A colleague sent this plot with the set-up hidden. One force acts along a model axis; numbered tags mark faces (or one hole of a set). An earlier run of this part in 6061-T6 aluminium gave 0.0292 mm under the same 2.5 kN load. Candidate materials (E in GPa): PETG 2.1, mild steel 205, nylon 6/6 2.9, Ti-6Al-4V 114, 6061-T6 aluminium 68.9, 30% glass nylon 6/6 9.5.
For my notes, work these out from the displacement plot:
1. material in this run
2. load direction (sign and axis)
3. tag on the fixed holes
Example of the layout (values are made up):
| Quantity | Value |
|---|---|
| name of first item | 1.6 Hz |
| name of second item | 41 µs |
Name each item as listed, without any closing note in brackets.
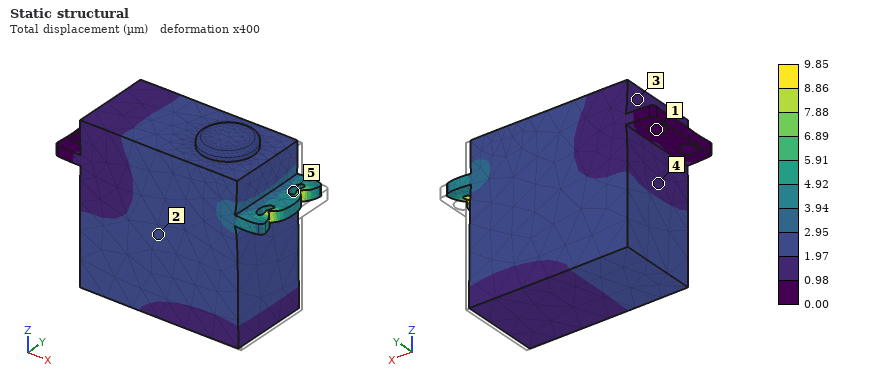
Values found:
| Quantity | Value |
|---|---|
| material in this run | mild steel |
| load direction | -X |
| tag on the fixed holes | 1 |
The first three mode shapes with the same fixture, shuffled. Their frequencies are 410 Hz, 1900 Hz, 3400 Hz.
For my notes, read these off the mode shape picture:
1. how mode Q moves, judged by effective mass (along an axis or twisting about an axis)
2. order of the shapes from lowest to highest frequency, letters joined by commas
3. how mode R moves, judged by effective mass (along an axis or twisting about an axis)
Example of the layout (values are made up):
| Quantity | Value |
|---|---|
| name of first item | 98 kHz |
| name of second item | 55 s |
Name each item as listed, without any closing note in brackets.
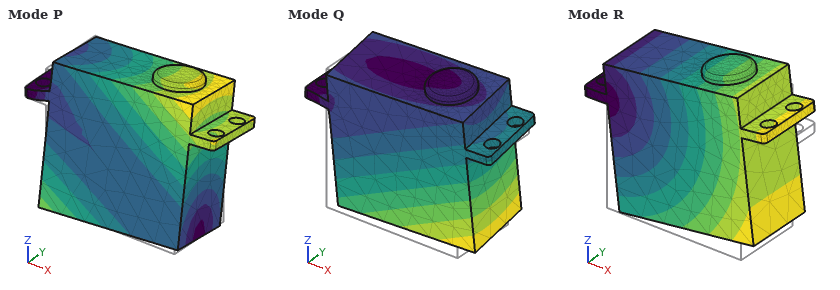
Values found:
| Quantity | Value |
|---|---|
| how mode Q moves, judged by effective mass | along Y |
| order of the shapes from lowest to highest frequency, letters joined by commas | R, Q, P |
| how mode R moves, judged by effective mass | along Z |
